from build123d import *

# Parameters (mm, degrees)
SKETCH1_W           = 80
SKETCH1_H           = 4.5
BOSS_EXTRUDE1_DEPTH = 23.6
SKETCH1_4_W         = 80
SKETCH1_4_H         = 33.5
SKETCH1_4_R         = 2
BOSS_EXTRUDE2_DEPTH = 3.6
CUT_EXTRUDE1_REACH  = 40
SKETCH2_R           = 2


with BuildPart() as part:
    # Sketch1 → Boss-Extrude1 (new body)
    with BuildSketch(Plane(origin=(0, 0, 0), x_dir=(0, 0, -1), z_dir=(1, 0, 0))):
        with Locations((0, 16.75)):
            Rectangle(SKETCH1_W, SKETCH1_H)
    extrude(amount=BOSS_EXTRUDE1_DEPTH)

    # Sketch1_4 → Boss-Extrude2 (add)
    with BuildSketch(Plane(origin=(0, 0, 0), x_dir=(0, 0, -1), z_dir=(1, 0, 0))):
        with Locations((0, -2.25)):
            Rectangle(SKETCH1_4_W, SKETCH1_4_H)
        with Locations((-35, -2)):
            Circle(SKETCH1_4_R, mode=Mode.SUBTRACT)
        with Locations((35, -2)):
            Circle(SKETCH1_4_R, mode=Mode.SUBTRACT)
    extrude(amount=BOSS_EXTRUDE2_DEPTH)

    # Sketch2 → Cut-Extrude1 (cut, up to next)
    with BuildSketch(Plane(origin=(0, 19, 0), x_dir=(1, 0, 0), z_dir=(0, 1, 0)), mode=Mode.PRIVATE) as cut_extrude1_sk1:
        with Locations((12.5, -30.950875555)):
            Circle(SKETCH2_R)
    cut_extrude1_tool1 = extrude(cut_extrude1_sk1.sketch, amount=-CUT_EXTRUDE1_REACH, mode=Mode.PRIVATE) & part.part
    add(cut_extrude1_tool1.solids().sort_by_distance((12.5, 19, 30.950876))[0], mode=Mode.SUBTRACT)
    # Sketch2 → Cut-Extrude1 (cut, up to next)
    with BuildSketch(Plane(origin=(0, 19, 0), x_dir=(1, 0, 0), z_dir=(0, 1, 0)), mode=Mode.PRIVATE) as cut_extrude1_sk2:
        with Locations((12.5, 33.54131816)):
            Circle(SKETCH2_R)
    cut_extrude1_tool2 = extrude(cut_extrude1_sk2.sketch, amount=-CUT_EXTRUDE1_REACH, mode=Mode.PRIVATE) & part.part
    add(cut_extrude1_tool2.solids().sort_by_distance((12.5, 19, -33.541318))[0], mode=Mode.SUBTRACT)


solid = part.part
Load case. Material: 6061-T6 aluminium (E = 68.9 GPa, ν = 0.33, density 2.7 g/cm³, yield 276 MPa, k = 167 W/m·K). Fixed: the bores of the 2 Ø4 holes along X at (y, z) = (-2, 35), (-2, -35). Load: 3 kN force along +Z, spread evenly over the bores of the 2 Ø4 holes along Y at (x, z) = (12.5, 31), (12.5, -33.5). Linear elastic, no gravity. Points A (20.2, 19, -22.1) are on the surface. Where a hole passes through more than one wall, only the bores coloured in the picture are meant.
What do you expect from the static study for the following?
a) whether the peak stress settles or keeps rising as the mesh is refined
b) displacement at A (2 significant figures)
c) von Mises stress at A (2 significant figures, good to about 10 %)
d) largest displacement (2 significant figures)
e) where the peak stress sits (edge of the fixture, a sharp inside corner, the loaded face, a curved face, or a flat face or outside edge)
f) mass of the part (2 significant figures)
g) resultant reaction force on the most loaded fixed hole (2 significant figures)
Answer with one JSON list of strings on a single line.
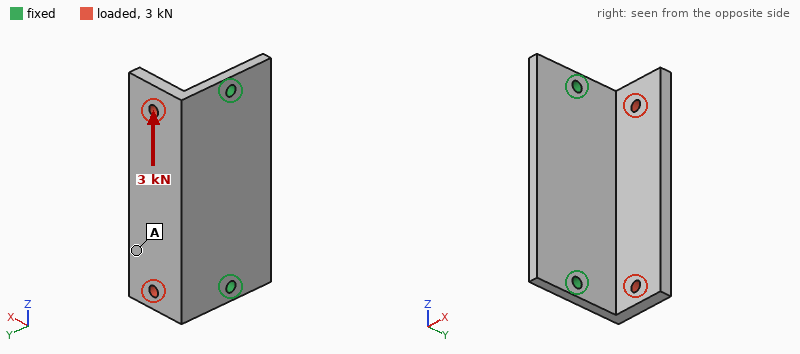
["keeps rising", "0.11 mm", "24 MPa", "0.17 mm", "edge of the fixture", "48 g", "1.8 kN"]
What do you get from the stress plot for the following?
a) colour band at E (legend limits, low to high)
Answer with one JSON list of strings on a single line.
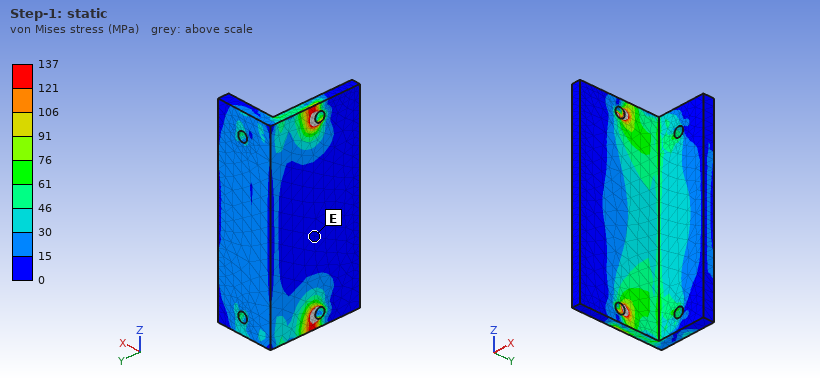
["0 to 15 MPa"]
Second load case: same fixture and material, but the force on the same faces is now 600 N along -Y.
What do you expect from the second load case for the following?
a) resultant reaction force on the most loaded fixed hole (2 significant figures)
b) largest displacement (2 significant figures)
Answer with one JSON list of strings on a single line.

["310 N", "0.22 mm"]
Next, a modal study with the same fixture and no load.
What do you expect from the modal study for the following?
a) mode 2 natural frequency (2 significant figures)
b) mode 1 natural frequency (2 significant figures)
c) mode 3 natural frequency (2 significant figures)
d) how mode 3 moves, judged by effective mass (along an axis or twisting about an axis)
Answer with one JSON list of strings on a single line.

["3600 Hz", "1700 Hz", "3900 Hz", "along X"]
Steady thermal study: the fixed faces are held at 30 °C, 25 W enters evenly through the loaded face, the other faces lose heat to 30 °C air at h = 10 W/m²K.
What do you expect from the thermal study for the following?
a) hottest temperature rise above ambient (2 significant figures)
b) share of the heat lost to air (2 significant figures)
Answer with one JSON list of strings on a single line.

["26 K", "5.0 %"]
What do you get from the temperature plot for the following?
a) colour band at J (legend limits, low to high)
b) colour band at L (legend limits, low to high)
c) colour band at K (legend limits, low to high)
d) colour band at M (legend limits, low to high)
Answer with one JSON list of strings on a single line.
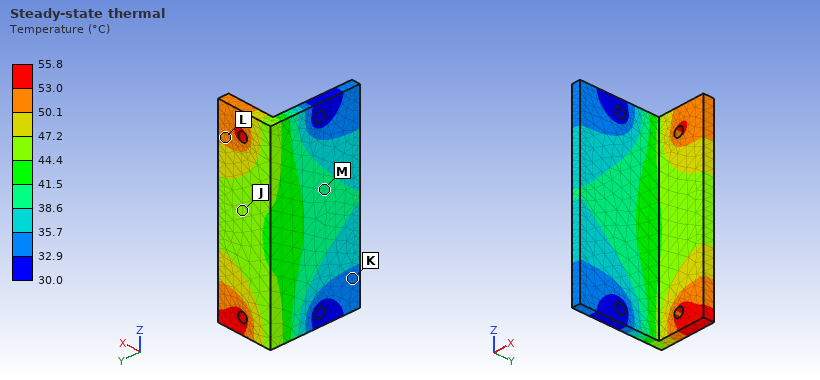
["44.4 to 47.2 °C", "50.1 to 53.0 °C", "32.9 to 35.7 °C", "38.6 to 41.5 °C"]
